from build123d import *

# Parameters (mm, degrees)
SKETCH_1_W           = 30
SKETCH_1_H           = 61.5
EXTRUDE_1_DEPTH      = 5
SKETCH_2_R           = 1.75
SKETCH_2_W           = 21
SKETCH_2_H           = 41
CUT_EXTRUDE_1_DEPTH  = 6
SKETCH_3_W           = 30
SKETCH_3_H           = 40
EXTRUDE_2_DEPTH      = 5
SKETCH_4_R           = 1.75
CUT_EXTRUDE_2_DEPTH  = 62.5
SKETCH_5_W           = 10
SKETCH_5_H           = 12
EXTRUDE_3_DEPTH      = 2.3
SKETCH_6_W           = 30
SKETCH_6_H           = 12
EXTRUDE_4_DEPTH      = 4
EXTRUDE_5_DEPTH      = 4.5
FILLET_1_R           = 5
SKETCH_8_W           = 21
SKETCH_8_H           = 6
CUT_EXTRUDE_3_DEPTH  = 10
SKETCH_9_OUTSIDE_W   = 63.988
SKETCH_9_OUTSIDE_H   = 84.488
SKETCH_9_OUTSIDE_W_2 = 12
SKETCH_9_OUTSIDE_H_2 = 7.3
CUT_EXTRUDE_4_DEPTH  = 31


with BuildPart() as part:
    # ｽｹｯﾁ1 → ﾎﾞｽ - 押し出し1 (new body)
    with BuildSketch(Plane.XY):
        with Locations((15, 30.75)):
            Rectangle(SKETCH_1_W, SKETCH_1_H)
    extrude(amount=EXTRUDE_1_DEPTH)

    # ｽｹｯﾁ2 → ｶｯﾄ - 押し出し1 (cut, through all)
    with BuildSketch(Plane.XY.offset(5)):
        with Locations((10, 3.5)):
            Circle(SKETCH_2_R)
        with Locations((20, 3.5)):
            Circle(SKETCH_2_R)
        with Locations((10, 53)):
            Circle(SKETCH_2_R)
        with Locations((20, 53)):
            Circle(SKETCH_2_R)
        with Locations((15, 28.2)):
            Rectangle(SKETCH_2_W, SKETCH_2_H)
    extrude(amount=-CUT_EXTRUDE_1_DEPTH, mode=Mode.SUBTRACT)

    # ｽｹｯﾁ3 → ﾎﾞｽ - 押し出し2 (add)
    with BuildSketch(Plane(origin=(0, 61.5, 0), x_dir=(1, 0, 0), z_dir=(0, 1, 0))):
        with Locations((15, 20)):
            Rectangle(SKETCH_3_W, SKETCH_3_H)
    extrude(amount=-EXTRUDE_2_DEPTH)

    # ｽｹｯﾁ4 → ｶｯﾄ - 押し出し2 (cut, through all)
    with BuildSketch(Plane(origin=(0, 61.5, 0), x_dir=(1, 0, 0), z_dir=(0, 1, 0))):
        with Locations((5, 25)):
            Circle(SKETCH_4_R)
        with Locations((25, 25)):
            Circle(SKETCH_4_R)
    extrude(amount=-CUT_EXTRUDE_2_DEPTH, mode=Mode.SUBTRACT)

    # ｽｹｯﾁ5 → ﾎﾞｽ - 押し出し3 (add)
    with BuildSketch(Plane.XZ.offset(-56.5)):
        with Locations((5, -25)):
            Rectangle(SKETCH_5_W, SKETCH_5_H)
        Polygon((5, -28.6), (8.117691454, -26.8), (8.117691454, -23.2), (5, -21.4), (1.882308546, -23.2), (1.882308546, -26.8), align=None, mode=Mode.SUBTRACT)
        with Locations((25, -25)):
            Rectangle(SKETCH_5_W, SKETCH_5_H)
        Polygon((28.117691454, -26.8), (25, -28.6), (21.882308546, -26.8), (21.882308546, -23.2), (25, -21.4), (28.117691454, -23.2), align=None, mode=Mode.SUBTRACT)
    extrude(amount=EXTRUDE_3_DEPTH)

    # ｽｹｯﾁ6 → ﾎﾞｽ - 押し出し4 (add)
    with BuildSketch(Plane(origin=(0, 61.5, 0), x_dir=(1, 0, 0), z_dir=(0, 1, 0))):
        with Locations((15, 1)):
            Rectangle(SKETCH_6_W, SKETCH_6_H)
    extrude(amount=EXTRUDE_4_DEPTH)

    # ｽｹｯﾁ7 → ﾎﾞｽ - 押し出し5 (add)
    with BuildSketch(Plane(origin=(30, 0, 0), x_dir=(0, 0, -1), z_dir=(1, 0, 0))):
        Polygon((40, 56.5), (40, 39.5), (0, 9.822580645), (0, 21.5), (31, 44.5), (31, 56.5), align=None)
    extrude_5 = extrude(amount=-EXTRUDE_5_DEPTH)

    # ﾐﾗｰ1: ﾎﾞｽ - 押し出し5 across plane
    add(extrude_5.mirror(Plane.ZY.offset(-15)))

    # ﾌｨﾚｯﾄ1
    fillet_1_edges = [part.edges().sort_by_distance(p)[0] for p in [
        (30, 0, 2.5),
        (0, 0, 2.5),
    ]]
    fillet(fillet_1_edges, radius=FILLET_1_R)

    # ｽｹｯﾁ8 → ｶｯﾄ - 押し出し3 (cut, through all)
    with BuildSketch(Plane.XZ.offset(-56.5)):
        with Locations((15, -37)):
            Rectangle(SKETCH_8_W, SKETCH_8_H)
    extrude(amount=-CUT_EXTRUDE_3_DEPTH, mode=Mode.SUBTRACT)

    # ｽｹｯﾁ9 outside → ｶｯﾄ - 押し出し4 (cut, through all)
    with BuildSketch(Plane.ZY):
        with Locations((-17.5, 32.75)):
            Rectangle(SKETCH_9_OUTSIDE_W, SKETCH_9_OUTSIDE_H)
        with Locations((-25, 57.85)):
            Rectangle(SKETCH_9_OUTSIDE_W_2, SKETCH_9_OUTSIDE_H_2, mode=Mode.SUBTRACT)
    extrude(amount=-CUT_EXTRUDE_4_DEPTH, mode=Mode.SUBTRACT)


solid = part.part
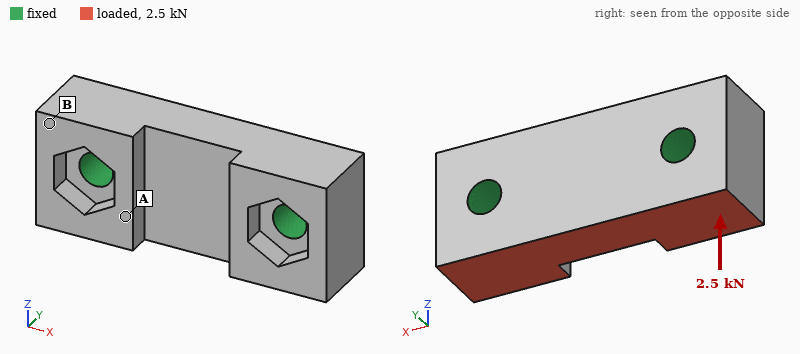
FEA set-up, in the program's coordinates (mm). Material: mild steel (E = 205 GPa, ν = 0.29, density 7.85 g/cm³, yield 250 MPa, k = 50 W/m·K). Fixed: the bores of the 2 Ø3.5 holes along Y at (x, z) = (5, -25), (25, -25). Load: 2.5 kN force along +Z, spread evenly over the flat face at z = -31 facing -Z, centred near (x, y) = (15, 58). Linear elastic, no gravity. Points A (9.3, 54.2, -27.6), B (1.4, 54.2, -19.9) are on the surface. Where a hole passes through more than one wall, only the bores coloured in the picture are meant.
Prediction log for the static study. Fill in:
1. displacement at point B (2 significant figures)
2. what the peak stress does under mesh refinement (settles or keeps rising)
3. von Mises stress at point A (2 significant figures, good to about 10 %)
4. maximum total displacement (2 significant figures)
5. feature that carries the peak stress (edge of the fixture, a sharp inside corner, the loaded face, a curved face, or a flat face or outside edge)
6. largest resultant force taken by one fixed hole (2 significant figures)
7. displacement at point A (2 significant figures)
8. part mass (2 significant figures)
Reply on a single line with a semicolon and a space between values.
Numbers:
0.49 µm; keeps rising; 16 MPa; 1.5 µm; edge of the fixture; 1.3 kN; 1.1 µm; 16 g
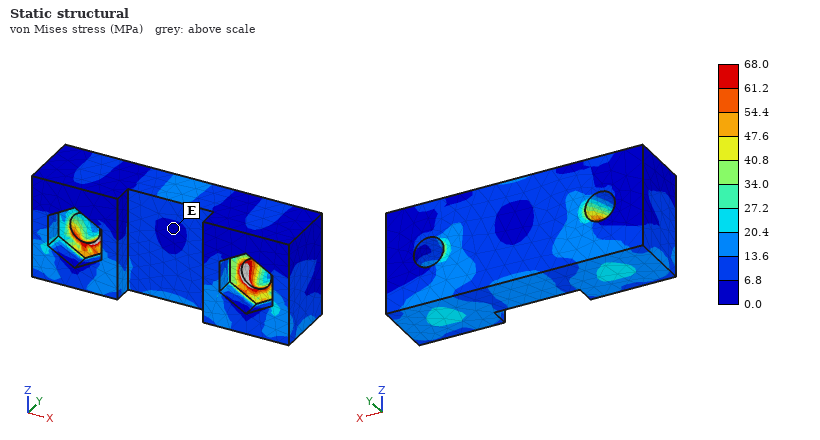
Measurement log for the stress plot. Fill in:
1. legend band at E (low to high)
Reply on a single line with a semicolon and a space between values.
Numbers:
0.0 to 6.8 MPa
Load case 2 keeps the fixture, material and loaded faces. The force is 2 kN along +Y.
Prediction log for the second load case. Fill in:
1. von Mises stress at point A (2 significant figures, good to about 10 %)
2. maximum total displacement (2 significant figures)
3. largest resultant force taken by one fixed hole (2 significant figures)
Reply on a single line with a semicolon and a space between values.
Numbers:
34 MPa; 5.8 µm; 1.0 kN
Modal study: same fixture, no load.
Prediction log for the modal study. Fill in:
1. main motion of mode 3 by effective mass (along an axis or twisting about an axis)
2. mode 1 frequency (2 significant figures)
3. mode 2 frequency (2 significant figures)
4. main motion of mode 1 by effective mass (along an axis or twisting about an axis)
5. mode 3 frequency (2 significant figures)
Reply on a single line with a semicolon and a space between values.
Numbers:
along Z; 49 kHz; 52 kHz; along Y; 58 kHz
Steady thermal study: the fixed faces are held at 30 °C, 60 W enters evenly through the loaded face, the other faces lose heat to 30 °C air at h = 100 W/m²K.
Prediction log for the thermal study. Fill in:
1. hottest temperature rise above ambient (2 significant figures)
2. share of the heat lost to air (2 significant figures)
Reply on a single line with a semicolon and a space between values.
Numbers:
55 K; 3.7 %
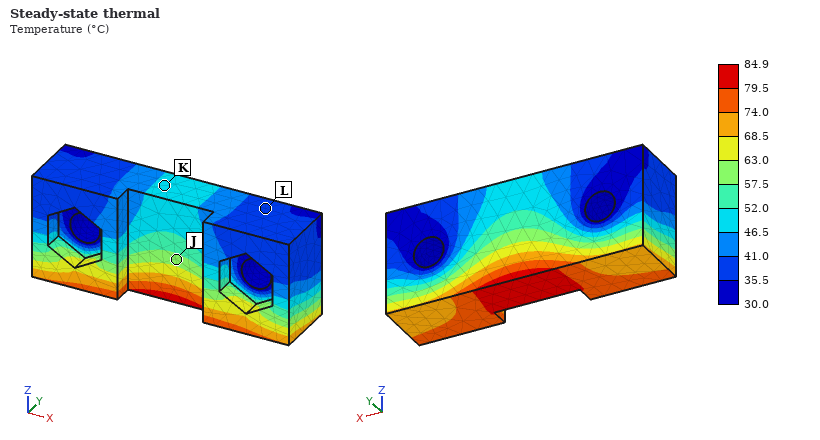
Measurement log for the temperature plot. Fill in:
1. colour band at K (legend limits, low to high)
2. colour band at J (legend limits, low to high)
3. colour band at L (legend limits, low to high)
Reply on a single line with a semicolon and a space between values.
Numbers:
46.5 to 52.0 °C; 57.5 to 63.0 °C; 35.5 to 41.0 °C
